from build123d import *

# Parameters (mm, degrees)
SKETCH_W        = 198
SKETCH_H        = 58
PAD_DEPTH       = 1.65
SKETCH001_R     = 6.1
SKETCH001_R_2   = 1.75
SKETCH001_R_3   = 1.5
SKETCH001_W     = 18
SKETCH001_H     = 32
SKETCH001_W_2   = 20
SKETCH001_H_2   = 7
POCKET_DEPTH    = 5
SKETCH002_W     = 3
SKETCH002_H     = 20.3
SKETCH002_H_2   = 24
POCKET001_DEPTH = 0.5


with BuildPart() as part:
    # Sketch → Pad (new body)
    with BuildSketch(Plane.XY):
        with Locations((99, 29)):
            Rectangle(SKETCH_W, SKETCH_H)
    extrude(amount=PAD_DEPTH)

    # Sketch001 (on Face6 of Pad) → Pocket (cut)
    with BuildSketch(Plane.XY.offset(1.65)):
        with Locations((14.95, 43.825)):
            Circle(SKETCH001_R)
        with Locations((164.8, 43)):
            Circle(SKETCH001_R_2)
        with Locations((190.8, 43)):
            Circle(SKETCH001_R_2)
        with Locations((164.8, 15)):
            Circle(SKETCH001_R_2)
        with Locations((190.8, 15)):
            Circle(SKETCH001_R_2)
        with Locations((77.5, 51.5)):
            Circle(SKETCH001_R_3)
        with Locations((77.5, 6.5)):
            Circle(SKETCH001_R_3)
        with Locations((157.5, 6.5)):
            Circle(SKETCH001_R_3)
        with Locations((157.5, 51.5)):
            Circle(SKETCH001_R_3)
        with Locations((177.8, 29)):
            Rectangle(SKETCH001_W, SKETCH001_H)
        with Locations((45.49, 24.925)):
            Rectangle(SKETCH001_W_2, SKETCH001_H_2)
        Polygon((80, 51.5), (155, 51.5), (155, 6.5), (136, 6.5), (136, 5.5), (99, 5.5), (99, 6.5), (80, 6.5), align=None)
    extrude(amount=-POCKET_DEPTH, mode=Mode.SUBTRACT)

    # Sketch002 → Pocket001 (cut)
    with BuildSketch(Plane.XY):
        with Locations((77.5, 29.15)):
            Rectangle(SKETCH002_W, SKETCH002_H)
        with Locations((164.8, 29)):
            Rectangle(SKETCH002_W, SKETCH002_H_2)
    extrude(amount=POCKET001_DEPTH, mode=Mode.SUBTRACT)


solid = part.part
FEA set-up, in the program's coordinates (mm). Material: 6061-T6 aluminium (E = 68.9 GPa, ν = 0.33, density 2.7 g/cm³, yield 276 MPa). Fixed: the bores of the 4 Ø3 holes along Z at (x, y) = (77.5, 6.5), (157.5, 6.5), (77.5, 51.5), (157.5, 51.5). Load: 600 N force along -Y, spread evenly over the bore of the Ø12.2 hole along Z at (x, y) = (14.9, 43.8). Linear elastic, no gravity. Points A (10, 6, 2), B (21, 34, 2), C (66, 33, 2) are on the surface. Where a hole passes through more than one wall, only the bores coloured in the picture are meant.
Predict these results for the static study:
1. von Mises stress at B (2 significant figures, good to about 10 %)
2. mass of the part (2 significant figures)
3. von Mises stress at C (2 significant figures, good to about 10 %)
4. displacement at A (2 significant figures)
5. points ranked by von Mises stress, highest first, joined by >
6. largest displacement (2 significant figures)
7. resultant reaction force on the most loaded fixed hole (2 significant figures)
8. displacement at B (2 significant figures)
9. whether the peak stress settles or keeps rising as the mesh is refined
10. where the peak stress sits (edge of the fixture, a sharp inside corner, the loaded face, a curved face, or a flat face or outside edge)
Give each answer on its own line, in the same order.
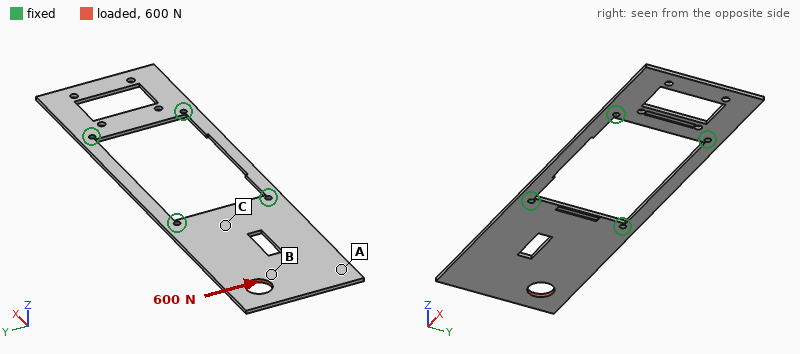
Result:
17 MPa
32 g
12 MPa
64 µm
B > C > A
76 µm
840 N
53 µm
keeps rising
edge of the fixture
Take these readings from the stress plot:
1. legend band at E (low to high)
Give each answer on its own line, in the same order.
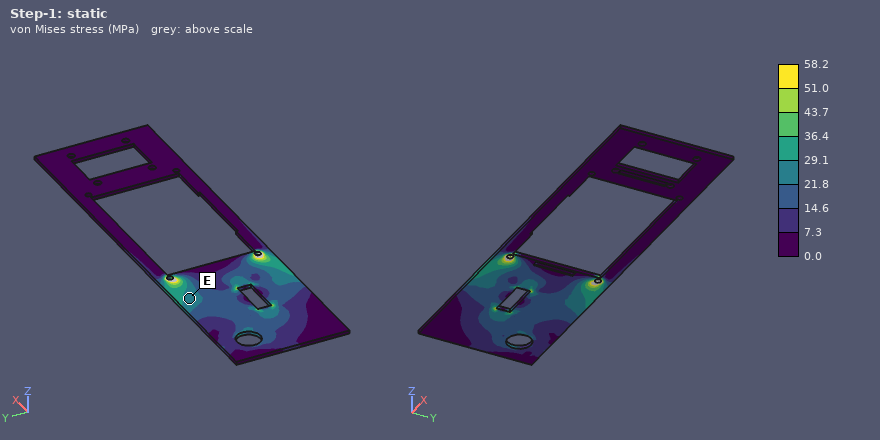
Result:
21.8 to 29.1 MPa
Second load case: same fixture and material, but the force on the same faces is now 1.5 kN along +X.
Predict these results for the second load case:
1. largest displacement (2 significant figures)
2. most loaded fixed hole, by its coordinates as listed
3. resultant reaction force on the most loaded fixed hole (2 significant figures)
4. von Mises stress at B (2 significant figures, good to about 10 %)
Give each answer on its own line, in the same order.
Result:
55 µm
(77.5, 51.5)
1.2 kN
28 MPa
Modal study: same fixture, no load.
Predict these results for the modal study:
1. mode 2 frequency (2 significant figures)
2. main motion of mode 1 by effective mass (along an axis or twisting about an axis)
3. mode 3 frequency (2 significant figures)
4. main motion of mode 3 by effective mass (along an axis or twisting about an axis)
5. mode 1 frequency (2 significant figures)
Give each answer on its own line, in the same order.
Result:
640 Hz
along Z
690 Hz
twisting about X
200 Hz
